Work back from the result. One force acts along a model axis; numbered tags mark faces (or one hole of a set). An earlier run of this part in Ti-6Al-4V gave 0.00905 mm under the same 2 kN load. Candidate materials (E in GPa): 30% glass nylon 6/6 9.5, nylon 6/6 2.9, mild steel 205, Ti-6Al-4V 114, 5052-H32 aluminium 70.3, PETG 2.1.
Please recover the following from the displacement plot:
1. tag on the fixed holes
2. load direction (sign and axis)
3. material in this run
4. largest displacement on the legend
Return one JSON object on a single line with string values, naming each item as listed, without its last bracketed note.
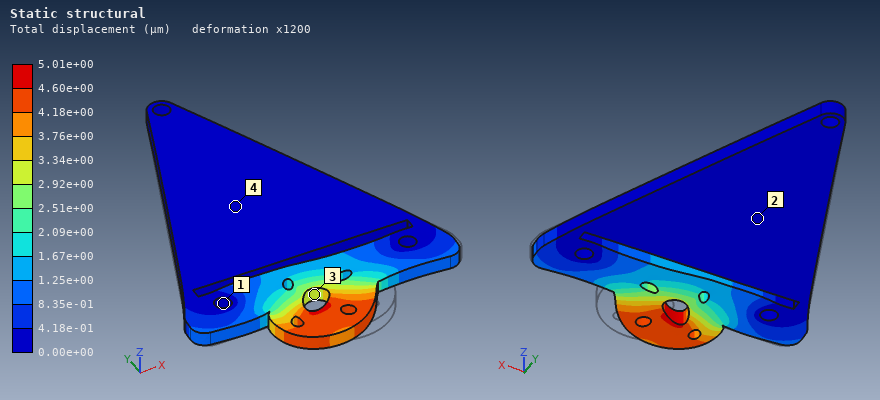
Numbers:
{"tag on the fixed holes": "1", "load direction": "-X", "material in this run": "mild steel", "largest displacement on the legend": "5.01e+00 µm"}
